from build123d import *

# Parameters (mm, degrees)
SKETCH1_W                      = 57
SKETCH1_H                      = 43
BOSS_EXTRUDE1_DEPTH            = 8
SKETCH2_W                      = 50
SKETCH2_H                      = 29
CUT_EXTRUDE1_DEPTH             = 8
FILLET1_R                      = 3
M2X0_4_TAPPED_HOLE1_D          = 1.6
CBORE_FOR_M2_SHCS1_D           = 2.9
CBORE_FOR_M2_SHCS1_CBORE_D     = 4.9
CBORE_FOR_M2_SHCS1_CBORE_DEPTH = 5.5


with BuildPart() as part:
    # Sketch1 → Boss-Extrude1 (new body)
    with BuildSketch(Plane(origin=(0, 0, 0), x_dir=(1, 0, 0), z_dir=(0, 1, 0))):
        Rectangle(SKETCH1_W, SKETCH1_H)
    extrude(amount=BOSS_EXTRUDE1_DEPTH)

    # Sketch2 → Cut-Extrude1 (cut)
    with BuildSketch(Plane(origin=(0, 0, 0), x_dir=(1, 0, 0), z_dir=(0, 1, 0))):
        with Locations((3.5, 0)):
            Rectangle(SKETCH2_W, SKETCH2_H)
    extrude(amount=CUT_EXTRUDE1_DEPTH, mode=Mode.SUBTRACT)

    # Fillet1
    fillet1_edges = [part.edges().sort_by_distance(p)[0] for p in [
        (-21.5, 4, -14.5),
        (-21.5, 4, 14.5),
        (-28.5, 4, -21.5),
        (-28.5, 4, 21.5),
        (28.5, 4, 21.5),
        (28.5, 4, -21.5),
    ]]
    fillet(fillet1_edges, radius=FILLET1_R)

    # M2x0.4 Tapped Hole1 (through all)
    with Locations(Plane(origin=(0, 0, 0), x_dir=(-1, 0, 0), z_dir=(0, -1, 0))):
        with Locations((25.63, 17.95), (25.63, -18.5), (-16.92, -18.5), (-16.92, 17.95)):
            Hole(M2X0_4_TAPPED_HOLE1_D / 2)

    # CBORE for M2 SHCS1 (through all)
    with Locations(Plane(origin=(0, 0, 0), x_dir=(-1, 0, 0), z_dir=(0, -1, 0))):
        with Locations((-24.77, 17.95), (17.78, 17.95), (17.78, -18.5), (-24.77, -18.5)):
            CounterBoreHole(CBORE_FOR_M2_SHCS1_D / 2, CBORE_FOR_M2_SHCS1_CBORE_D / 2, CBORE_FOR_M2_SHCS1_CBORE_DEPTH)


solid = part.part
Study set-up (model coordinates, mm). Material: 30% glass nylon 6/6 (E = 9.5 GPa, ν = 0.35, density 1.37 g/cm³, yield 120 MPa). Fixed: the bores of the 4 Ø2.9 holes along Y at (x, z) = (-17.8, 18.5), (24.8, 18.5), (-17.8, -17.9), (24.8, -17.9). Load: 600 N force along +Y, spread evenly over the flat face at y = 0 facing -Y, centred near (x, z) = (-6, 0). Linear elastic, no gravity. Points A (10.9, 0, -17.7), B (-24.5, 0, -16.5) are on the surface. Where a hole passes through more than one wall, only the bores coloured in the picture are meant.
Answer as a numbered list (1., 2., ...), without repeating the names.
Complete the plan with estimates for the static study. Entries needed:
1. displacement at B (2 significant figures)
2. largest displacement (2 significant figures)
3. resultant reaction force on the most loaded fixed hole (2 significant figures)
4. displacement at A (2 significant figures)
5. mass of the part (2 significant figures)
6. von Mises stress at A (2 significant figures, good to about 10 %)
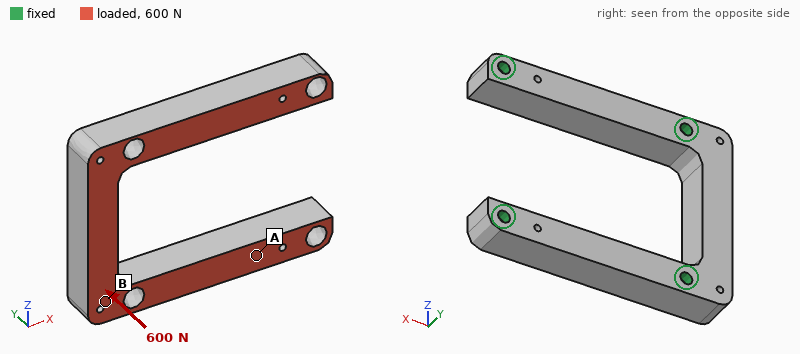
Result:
1. 19 µm
2. 45 µm
3. 220 N
4. 24 µm
5. 10 g
6. 5.6 MPa
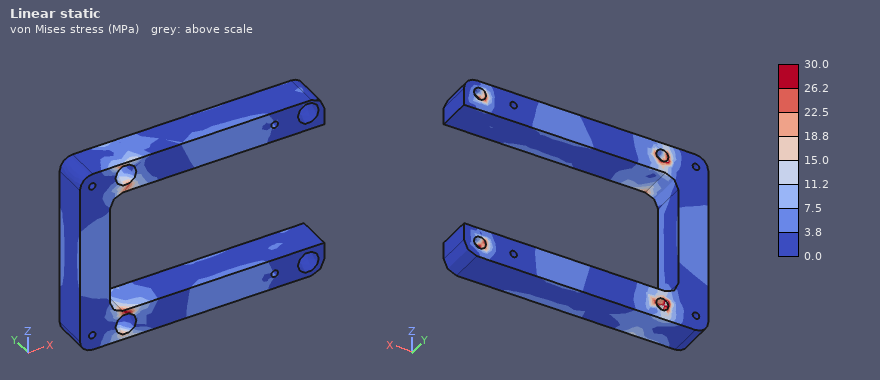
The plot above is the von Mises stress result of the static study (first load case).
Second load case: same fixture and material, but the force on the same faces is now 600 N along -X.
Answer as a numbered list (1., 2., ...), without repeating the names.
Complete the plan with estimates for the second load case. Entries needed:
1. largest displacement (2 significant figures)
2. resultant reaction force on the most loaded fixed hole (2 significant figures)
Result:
1. 63 µm
2. 170 N
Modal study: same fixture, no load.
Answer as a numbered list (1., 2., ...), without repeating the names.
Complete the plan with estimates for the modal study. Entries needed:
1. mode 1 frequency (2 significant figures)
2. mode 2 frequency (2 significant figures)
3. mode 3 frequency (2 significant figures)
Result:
1. 5800 Hz
2. 6400 Hz
3. 6600 Hz
